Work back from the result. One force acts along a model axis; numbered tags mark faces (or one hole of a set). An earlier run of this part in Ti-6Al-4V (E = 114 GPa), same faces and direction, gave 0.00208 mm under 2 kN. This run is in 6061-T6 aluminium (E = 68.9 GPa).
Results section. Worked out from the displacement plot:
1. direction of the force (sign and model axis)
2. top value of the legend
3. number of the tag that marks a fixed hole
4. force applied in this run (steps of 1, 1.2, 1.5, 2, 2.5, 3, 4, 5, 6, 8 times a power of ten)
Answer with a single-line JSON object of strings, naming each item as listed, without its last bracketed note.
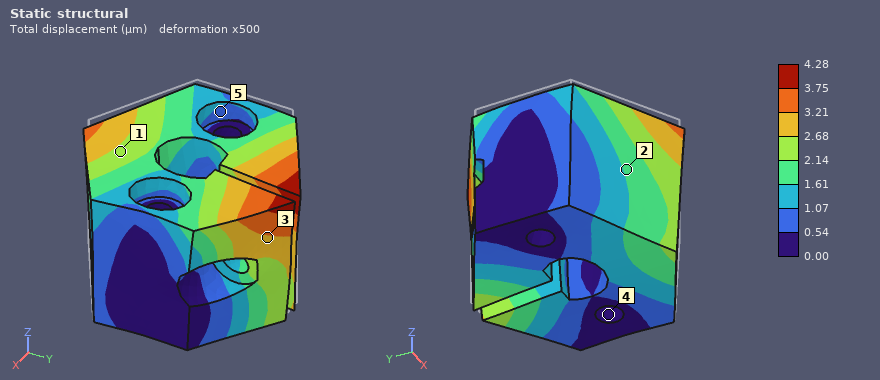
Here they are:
{"direction of the force": "-Z", "top value of the legend": "4.28 µm", "number of the tag that marks a fixed hole": "4", "force applied in this run": "2.5 kN"}
